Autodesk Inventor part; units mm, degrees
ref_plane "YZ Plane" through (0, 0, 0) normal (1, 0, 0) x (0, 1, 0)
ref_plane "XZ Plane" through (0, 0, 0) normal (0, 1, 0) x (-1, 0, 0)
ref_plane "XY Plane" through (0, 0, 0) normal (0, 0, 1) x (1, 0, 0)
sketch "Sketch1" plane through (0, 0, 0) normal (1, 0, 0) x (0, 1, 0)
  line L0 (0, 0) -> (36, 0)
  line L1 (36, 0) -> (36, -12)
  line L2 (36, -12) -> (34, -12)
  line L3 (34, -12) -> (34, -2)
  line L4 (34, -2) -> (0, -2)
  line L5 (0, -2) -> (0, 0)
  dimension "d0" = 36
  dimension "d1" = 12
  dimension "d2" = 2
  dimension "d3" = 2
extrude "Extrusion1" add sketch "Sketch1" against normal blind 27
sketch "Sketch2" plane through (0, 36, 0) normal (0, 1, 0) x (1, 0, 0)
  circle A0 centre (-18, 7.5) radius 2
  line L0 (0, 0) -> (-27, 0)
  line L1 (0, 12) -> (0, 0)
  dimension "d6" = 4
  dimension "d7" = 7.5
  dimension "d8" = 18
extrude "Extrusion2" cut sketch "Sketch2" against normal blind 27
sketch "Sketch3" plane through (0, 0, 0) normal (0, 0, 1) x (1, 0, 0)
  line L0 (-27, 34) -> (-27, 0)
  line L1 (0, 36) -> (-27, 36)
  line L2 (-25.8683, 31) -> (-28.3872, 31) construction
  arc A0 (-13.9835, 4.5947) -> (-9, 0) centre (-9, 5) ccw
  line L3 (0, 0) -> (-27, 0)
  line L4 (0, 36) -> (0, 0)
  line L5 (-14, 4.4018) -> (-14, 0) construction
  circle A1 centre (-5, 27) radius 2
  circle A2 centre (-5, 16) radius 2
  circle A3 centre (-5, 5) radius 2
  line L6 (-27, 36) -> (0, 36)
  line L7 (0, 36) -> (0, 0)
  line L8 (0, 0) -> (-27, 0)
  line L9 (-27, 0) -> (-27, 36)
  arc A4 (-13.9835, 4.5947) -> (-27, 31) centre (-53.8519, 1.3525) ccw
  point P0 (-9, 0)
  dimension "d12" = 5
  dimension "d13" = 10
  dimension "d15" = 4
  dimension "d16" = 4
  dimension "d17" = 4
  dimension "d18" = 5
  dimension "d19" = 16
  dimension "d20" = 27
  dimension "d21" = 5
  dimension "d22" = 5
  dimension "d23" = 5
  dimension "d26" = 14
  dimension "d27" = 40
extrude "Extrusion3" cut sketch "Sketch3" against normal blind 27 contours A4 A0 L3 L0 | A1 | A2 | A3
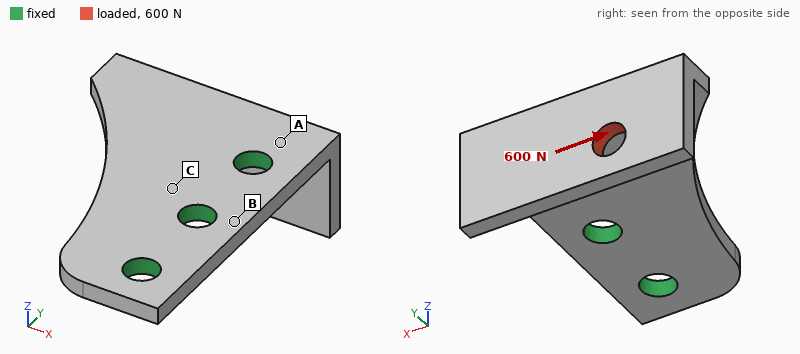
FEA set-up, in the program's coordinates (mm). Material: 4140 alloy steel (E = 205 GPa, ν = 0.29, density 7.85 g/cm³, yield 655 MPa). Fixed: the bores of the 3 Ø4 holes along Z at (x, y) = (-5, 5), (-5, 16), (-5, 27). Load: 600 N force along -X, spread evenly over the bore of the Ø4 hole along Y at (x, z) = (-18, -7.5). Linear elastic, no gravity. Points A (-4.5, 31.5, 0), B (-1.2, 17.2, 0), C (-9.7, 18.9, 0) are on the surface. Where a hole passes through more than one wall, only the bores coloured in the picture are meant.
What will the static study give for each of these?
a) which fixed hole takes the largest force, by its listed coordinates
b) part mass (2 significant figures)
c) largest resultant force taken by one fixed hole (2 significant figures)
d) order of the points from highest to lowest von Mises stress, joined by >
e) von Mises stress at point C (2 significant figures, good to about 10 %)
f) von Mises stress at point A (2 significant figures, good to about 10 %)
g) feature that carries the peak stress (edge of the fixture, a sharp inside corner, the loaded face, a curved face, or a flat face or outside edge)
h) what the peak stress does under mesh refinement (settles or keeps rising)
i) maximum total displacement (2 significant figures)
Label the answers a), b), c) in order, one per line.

a) (-5, 27)
b) 14 g
c) 790 N
d) A > C > B
e) 80 MPa
f) 190 MPa
g) edge of the fixture
h) keeps rising
i) 0.15 mm
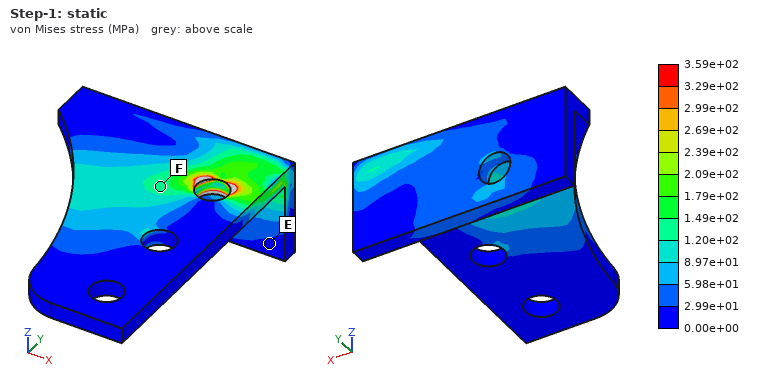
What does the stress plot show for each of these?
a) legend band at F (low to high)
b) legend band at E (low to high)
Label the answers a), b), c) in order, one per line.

a) 1.20e+02 to 1.49e+02 MPa
b) 0.00e+00 to 2.99e+01 MPa
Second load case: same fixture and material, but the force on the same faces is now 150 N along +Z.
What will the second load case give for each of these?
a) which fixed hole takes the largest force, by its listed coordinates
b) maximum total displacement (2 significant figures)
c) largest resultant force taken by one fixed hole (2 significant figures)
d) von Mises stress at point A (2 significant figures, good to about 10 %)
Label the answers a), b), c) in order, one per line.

a) (-5, 27)
b) 86 µm
c) 180 N
d) 120 MPa
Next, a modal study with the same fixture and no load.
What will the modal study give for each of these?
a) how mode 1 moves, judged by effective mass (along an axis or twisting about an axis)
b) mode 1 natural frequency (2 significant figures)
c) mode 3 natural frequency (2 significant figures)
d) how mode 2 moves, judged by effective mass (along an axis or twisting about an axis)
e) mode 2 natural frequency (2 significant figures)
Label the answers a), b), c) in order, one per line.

a) along Z
b) 3700 Hz
c) 12 kHz
d) along Y
e) 6600 Hz
